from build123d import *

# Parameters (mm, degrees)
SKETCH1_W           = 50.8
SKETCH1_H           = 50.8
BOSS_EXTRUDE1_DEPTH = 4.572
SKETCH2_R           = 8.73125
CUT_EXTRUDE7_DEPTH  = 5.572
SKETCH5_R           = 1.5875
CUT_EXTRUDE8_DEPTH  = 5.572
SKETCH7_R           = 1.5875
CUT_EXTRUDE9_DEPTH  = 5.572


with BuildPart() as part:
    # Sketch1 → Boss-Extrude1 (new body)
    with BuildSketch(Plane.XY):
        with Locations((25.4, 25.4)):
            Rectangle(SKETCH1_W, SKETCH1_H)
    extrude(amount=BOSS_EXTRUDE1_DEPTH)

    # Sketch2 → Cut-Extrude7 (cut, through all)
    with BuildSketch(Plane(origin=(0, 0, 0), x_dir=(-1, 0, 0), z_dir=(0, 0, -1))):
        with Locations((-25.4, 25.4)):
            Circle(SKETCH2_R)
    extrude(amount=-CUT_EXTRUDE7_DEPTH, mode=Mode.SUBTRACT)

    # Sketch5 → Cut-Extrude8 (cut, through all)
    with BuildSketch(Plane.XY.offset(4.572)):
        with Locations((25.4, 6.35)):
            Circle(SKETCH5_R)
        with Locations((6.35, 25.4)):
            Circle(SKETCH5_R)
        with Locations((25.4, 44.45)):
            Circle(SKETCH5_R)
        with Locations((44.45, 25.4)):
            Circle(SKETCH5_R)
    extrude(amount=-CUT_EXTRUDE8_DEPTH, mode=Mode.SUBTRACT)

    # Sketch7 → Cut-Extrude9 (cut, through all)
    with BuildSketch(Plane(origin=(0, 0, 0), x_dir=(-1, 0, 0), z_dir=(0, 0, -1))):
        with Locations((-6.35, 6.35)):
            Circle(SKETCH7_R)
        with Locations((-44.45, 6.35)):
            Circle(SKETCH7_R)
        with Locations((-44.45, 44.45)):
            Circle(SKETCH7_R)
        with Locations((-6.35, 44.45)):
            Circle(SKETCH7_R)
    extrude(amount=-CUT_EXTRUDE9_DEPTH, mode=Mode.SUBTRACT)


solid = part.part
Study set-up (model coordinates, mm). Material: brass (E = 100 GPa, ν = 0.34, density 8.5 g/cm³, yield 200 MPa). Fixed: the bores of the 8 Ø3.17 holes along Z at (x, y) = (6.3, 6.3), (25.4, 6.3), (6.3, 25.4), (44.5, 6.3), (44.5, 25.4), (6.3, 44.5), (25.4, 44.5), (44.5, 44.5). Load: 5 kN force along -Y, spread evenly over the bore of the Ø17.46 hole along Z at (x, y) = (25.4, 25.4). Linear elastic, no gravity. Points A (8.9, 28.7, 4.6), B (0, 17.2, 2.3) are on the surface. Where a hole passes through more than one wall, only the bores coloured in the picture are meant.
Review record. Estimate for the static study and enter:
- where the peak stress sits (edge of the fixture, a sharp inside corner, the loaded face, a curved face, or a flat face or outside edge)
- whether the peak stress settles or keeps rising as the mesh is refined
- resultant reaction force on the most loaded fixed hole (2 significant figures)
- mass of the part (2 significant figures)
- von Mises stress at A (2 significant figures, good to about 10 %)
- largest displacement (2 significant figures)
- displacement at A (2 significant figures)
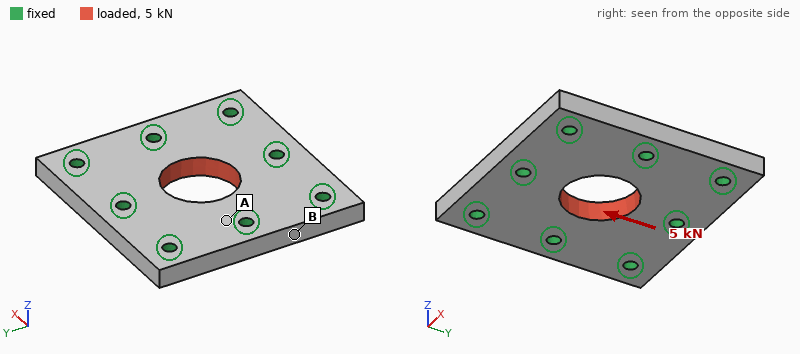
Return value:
edge of the fixture
keeps rising
1.2 kN
89 g
10 MPa
3.1 µm
0.60 µm
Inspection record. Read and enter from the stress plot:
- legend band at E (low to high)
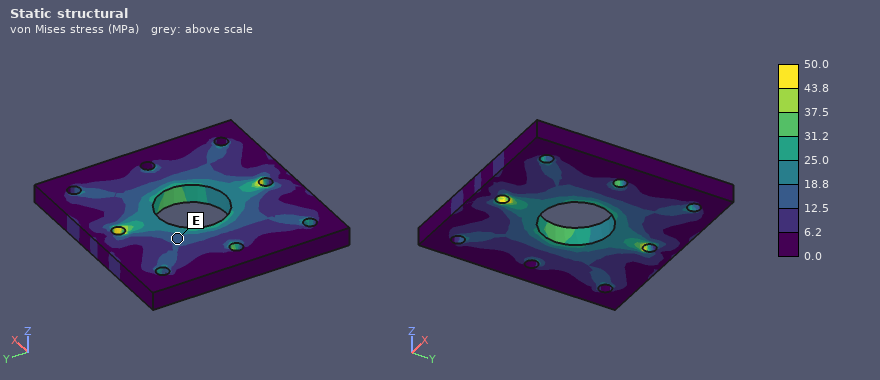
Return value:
12.5 to 18.8 MPa
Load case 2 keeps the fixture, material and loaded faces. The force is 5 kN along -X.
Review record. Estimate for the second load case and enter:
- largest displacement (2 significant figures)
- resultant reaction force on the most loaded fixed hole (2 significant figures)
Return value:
3.1 µm
1.2 kN
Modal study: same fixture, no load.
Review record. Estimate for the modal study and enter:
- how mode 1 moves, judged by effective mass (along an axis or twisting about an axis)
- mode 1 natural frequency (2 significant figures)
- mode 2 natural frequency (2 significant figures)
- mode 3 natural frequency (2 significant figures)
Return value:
along Z
19 kHz
24 kHz
24 kHz
